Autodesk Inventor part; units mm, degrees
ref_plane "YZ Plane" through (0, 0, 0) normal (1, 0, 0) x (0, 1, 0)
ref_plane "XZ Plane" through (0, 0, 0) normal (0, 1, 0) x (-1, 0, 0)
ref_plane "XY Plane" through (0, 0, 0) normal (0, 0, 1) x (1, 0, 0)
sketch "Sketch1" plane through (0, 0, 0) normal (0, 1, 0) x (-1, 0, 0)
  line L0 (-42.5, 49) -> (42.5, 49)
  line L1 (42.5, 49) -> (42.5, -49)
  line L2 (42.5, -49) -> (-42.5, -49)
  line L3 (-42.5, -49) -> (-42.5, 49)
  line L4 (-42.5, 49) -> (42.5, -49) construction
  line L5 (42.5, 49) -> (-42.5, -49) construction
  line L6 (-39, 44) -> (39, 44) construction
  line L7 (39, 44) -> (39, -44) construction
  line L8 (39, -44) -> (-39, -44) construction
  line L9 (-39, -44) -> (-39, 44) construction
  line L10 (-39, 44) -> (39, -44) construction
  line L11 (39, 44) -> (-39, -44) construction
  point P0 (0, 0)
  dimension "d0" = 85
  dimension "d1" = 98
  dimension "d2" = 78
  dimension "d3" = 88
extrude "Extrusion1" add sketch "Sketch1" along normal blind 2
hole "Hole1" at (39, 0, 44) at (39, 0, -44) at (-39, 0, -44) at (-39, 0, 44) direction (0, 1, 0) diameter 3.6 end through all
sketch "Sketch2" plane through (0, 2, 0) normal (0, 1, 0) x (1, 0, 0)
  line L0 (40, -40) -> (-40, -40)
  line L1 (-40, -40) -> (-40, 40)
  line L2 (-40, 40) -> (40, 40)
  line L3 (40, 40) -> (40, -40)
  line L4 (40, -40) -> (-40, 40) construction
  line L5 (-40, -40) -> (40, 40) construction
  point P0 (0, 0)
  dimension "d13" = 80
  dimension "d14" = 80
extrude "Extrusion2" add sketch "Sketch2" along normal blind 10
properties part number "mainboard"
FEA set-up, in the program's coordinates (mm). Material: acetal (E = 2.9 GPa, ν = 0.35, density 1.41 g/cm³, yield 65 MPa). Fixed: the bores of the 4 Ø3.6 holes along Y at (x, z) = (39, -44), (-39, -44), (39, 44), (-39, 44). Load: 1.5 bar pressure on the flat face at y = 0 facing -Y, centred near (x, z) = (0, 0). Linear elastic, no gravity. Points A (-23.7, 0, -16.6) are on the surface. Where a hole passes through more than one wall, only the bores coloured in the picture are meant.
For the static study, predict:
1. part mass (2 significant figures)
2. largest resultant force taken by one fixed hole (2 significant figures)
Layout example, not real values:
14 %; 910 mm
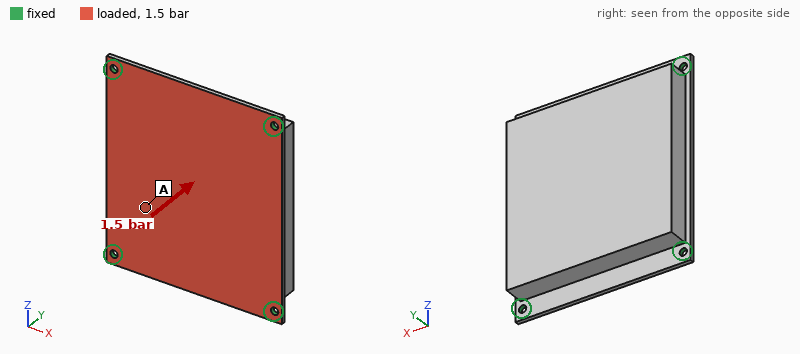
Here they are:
110 g; 460 N
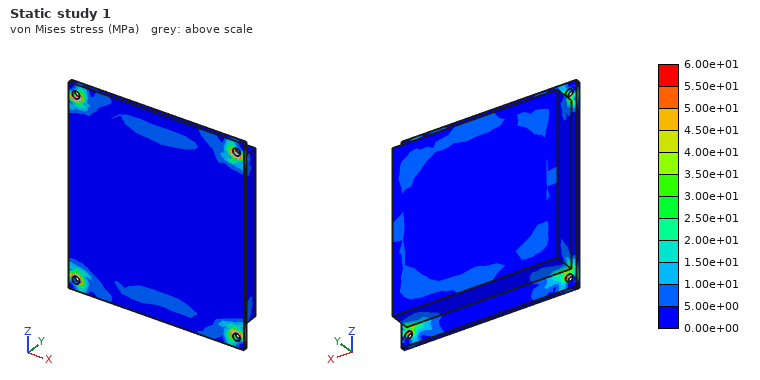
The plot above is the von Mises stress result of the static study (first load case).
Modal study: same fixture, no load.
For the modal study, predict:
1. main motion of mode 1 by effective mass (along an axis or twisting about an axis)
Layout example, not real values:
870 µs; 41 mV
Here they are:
along Y
